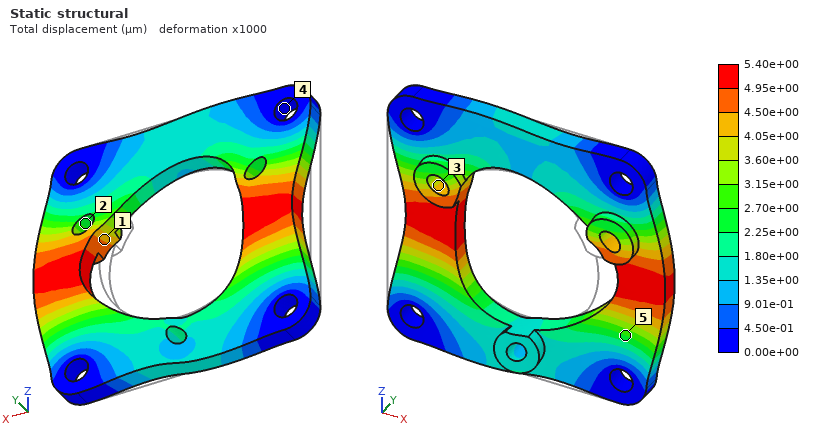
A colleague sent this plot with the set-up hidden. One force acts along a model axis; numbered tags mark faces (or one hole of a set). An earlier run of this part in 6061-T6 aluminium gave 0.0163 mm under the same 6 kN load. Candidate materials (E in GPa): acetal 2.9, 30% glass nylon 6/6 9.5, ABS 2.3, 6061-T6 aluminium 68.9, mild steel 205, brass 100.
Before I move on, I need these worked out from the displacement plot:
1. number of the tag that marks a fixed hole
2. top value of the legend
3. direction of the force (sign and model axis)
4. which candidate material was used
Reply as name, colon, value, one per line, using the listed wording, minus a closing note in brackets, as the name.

number of the tag that marks a fixed hole: 4
top value of the legend: 5.40e+00 µm
direction of the force: +X
which candidate material was used: mild steel
